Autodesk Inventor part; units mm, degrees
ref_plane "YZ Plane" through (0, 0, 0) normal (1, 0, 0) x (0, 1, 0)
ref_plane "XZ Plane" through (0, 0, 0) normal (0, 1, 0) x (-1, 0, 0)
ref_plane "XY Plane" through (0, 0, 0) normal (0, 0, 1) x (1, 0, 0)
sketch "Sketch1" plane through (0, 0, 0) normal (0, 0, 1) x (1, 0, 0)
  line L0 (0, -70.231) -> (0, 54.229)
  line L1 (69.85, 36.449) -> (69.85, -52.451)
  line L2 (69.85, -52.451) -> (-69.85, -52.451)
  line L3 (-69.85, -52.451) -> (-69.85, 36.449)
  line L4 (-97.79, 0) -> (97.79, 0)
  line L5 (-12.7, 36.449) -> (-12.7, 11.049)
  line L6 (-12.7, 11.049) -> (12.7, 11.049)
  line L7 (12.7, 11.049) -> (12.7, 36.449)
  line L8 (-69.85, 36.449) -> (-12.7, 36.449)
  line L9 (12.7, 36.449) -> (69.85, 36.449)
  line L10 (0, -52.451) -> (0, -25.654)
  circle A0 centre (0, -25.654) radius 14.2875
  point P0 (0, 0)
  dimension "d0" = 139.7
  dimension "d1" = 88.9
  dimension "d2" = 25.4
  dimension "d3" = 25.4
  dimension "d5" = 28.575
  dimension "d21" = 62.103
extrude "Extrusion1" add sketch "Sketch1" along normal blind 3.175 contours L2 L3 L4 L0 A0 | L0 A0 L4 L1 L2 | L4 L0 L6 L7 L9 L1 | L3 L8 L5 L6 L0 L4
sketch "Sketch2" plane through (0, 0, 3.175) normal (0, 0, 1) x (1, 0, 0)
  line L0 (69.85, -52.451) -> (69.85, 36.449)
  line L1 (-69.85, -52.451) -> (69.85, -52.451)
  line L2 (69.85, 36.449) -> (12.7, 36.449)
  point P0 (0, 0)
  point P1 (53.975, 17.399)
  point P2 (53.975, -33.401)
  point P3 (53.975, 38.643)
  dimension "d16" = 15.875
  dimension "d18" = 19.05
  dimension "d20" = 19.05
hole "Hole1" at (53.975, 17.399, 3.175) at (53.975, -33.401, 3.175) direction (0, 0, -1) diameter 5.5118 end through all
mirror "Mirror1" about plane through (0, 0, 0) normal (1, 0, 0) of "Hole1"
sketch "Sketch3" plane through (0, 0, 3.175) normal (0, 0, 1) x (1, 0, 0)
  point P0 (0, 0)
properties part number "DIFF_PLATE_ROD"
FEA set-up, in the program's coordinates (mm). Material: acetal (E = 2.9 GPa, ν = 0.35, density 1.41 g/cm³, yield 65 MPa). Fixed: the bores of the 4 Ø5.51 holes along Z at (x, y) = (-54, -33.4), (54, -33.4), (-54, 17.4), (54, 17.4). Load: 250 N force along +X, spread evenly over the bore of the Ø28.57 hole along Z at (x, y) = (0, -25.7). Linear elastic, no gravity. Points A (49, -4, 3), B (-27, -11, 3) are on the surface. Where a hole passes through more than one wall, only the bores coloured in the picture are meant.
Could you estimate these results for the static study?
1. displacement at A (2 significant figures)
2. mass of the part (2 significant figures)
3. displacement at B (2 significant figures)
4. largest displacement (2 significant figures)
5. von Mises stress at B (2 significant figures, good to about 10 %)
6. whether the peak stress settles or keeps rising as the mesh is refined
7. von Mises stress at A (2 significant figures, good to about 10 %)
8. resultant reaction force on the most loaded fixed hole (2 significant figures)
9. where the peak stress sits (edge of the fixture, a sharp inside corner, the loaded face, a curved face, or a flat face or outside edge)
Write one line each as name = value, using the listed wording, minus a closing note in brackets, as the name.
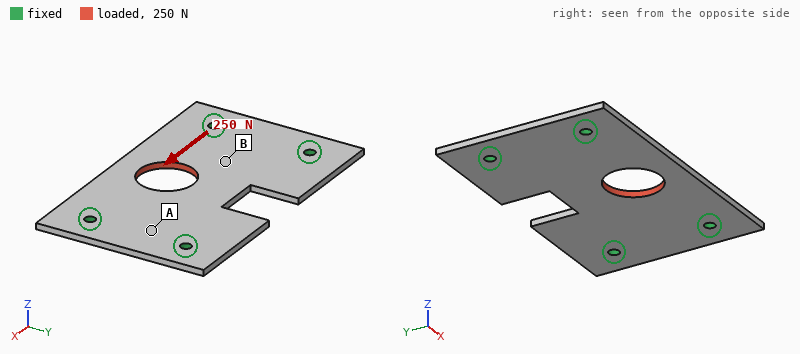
displacement at A = 4.9 µm
mass of the part = 49 g
displacement at B = 8.1 µm
largest displacement = 18 µm
von Mises stress at B = 0.54 MPa
whether the peak stress settles or keeps rising as the mesh is refined = keeps rising
von Mises stress at A = 0.26 MPa
resultant reaction force on the most loaded fixed hole = 88 N
where the peak stress sits = edge of the fixture
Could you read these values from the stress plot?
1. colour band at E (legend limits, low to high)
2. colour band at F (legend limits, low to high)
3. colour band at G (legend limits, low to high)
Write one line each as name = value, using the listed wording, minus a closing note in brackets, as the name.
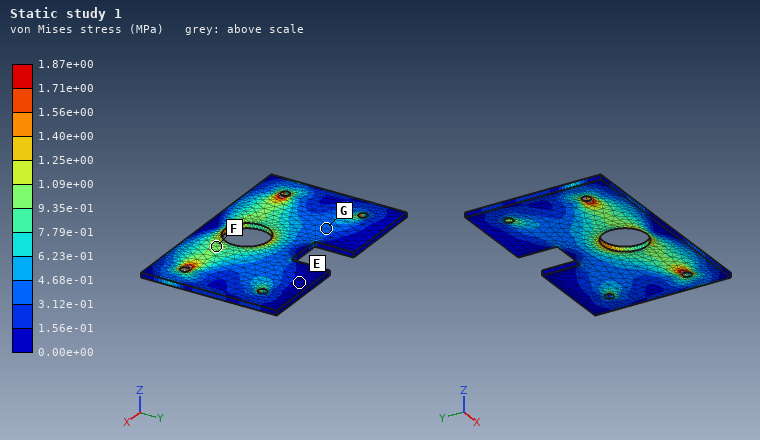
colour band at E = 0.00e+00 to 1.56e-01 MPa
colour band at F = 9.35e-01 to 1.09e+00 MPa
colour band at G = 3.12e-01 to 4.68e-01 MPa
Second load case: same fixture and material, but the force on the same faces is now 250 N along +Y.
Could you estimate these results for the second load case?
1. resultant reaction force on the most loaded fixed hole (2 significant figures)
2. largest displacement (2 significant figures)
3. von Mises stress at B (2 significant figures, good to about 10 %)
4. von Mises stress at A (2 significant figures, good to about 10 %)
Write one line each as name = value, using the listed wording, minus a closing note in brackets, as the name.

resultant reaction force on the most loaded fixed hole = 98 N
largest displacement = 47 µm
von Mises stress at B = 1.3 MPa
von Mises stress at A = 0.88 MPa
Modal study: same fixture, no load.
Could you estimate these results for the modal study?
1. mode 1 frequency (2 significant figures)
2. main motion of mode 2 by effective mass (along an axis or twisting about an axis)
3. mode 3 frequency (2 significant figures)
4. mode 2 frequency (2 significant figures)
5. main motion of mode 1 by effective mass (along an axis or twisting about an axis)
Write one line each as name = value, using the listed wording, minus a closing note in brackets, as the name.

mode 1 frequency = 400 Hz
main motion of mode 2 by effective mass = twisting about X
mode 3 frequency = 780 Hz
mode 2 frequency = 540 Hz
main motion of mode 1 by effective mass = along Z
